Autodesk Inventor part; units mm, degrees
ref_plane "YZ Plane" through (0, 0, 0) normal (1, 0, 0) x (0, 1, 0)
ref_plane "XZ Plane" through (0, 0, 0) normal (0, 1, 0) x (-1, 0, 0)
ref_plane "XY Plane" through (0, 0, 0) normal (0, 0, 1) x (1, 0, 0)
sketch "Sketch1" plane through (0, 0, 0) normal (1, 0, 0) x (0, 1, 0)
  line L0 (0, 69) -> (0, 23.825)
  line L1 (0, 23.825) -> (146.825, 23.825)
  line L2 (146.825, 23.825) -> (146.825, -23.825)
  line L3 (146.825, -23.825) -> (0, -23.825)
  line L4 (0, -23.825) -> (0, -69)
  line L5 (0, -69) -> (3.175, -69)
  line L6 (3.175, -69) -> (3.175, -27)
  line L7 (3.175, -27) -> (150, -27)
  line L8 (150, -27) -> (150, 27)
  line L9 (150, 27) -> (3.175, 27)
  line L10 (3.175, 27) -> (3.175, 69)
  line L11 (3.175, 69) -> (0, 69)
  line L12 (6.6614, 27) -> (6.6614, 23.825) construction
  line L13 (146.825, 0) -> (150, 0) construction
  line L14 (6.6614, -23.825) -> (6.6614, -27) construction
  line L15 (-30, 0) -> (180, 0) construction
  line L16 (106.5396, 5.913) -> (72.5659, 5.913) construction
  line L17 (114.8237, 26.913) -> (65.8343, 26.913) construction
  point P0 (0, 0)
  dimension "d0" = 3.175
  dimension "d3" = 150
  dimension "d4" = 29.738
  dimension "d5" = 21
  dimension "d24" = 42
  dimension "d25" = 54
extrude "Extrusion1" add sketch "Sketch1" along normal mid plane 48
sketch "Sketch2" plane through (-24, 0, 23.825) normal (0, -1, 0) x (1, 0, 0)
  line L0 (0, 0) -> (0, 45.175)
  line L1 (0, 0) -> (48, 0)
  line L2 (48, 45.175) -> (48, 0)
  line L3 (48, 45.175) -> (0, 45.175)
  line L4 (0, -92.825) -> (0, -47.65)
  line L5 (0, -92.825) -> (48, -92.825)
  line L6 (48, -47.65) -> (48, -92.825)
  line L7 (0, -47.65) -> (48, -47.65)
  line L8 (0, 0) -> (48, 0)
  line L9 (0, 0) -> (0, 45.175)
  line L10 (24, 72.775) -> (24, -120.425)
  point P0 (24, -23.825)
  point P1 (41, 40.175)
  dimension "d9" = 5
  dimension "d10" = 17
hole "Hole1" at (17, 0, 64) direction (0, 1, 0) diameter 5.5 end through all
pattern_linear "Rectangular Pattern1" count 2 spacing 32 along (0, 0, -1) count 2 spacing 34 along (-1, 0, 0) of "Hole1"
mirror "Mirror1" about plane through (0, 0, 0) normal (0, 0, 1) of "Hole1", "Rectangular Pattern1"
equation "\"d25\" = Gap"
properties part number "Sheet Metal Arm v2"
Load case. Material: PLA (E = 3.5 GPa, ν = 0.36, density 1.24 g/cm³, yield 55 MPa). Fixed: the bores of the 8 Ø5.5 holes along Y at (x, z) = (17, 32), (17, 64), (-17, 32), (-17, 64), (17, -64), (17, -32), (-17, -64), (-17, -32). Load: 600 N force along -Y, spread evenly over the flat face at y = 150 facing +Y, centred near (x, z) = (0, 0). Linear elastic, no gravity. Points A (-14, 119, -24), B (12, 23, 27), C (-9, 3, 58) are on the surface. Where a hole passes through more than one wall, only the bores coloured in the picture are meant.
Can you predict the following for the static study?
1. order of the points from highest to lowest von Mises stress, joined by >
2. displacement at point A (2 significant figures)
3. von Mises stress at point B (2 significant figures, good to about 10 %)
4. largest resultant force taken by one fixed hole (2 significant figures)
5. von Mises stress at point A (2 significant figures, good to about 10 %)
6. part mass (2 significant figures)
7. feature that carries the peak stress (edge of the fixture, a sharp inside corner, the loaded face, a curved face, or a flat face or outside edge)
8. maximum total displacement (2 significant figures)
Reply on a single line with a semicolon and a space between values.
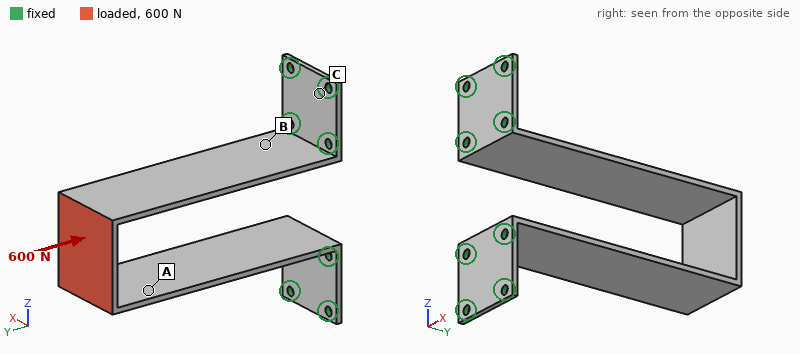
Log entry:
A > B > C; 1.4 mm; 5.8 MPa; 150 N; 10 MPa; 81 g; the loaded face; 1.7 mm
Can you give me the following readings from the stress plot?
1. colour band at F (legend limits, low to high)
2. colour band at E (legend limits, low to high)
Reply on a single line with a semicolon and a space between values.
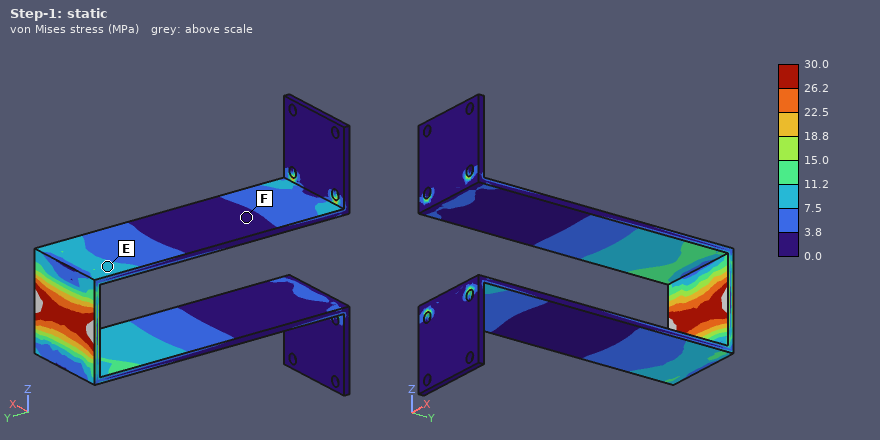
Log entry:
0.0 to 3.8 MPa; 7.5 to 11.2 MPa
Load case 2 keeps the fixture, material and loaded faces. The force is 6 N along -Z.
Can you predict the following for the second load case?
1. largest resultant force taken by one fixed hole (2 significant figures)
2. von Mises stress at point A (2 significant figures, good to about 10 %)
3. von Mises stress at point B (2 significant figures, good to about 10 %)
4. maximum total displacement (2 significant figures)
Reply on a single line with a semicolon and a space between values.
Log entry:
4.2 N; 1.6 MPa; 1.9 MPa; 2.0 mm
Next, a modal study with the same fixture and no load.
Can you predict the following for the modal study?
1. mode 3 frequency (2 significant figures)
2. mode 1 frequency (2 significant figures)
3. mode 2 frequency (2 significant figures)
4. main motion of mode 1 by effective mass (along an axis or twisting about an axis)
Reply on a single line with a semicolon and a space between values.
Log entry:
280 Hz; 50 Hz; 210 Hz; along Z
